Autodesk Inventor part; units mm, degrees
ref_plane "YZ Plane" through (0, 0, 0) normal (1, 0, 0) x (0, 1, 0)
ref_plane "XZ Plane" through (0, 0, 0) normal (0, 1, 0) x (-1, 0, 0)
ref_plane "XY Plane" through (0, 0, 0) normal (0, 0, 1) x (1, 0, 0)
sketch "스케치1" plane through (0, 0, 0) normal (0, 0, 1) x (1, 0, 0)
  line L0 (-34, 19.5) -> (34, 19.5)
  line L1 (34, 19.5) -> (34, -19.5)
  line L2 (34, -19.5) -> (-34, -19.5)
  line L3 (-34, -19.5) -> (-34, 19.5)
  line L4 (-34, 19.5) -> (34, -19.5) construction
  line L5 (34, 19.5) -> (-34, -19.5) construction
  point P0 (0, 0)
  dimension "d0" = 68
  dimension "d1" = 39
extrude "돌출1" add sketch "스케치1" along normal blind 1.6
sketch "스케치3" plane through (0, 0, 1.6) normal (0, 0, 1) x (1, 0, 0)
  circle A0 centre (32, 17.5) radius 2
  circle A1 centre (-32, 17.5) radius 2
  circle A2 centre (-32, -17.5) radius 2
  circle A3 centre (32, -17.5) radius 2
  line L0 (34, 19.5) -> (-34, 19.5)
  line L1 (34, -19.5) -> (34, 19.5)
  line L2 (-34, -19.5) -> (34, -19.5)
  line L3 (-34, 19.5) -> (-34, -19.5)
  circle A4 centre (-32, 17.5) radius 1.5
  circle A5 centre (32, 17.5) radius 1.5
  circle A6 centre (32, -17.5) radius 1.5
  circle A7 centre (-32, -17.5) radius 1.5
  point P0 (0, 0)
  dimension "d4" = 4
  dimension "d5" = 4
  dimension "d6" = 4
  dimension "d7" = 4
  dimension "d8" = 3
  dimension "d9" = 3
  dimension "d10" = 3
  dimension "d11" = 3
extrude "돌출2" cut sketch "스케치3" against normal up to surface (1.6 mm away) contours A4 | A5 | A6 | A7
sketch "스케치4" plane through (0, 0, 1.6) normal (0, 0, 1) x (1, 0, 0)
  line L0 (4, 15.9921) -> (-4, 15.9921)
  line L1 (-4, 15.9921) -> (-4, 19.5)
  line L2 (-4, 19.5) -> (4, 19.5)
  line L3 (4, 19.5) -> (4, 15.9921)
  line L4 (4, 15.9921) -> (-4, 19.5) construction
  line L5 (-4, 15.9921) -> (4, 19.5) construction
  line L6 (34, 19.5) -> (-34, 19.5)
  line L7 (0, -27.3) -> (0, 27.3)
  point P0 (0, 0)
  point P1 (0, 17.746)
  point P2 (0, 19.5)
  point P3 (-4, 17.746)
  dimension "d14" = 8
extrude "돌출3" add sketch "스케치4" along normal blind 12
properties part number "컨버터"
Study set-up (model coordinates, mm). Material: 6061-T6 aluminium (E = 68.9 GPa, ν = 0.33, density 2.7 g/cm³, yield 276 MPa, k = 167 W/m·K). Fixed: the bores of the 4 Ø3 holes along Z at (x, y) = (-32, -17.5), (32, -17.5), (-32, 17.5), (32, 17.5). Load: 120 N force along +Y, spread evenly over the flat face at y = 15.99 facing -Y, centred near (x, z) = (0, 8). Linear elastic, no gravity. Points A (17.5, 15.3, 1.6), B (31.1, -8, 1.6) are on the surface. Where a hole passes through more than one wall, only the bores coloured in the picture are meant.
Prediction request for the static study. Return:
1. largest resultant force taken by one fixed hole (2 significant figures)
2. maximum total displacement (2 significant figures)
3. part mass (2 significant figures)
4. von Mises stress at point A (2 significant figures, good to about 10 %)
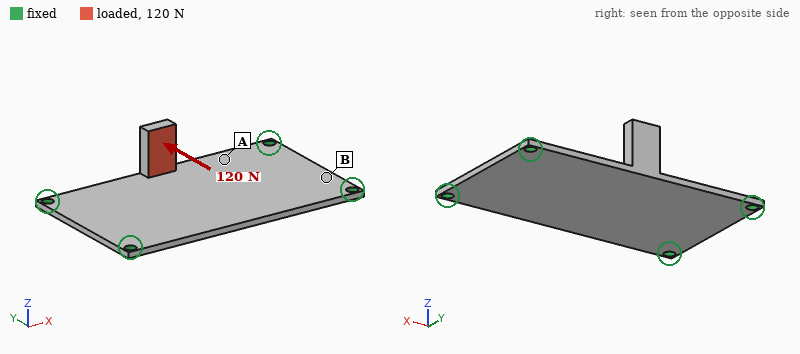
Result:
45 N
0.26 mm
12 g
36 MPa
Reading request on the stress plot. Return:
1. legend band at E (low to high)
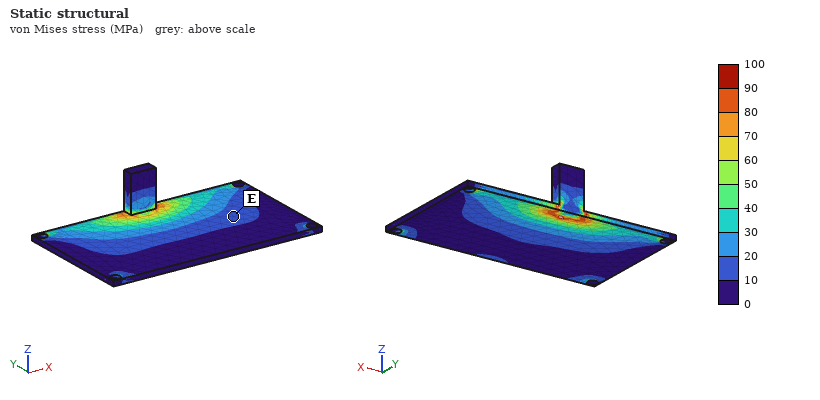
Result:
10 to 20 MPa
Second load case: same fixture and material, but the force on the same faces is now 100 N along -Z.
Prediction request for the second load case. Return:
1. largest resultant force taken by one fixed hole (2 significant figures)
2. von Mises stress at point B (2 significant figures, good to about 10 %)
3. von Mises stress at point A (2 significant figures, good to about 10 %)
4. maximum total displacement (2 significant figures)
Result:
50 N
21 MPa
45 MPa
0.34 mm
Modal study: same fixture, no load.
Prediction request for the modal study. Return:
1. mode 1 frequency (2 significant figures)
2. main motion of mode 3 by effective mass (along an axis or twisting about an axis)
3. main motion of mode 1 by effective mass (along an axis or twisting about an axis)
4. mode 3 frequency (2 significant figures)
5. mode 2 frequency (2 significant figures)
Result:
1600 Hz
twisting about Y
along Z
4400 Hz
2500 Hz
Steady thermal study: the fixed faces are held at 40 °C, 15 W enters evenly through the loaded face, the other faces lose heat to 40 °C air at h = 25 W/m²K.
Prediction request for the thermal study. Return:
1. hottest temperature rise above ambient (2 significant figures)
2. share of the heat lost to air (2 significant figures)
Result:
68 K
15 %
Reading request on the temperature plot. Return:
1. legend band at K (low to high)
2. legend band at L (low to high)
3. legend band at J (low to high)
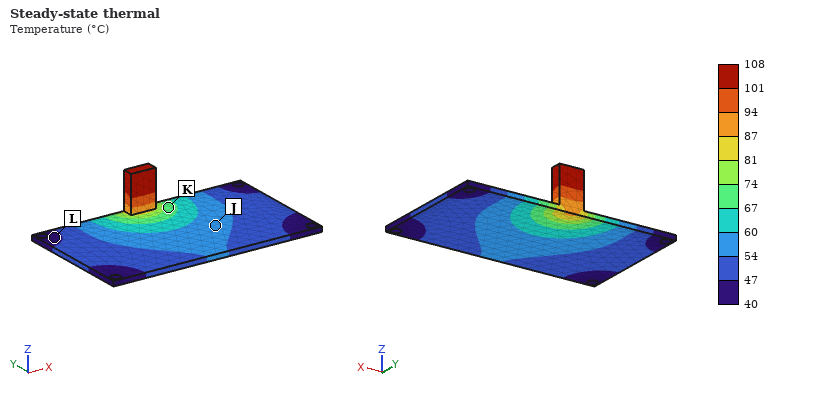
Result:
67 to 74 °C
40 to 47 °C
54 to 60 °C
